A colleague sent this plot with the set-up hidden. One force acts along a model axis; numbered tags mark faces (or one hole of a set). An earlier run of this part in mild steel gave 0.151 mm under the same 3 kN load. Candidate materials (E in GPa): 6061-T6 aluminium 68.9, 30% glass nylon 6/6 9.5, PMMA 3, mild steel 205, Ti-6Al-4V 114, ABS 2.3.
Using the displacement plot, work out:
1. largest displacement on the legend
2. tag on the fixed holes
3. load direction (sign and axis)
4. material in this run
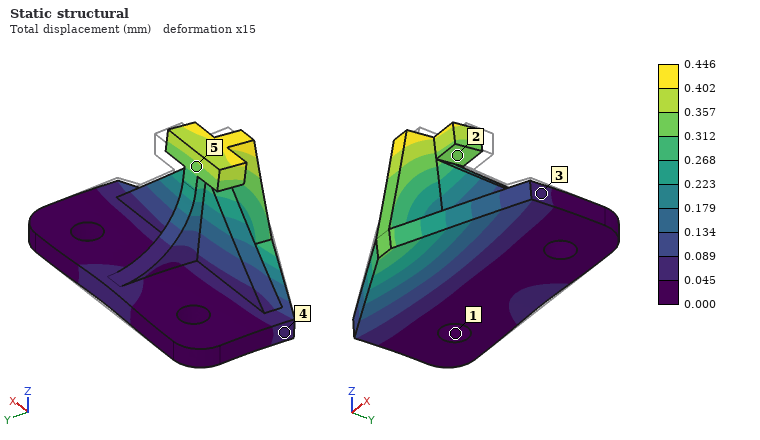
0.446 mm
1
-Y
6061-T6 aluminium
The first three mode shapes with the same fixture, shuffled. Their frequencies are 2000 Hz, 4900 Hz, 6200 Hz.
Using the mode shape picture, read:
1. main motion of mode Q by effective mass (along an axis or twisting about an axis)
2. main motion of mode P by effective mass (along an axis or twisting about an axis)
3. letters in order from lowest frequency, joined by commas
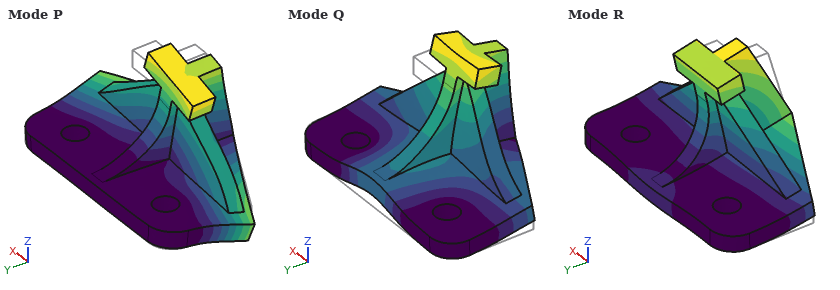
along Z
along X
R, P, Q
